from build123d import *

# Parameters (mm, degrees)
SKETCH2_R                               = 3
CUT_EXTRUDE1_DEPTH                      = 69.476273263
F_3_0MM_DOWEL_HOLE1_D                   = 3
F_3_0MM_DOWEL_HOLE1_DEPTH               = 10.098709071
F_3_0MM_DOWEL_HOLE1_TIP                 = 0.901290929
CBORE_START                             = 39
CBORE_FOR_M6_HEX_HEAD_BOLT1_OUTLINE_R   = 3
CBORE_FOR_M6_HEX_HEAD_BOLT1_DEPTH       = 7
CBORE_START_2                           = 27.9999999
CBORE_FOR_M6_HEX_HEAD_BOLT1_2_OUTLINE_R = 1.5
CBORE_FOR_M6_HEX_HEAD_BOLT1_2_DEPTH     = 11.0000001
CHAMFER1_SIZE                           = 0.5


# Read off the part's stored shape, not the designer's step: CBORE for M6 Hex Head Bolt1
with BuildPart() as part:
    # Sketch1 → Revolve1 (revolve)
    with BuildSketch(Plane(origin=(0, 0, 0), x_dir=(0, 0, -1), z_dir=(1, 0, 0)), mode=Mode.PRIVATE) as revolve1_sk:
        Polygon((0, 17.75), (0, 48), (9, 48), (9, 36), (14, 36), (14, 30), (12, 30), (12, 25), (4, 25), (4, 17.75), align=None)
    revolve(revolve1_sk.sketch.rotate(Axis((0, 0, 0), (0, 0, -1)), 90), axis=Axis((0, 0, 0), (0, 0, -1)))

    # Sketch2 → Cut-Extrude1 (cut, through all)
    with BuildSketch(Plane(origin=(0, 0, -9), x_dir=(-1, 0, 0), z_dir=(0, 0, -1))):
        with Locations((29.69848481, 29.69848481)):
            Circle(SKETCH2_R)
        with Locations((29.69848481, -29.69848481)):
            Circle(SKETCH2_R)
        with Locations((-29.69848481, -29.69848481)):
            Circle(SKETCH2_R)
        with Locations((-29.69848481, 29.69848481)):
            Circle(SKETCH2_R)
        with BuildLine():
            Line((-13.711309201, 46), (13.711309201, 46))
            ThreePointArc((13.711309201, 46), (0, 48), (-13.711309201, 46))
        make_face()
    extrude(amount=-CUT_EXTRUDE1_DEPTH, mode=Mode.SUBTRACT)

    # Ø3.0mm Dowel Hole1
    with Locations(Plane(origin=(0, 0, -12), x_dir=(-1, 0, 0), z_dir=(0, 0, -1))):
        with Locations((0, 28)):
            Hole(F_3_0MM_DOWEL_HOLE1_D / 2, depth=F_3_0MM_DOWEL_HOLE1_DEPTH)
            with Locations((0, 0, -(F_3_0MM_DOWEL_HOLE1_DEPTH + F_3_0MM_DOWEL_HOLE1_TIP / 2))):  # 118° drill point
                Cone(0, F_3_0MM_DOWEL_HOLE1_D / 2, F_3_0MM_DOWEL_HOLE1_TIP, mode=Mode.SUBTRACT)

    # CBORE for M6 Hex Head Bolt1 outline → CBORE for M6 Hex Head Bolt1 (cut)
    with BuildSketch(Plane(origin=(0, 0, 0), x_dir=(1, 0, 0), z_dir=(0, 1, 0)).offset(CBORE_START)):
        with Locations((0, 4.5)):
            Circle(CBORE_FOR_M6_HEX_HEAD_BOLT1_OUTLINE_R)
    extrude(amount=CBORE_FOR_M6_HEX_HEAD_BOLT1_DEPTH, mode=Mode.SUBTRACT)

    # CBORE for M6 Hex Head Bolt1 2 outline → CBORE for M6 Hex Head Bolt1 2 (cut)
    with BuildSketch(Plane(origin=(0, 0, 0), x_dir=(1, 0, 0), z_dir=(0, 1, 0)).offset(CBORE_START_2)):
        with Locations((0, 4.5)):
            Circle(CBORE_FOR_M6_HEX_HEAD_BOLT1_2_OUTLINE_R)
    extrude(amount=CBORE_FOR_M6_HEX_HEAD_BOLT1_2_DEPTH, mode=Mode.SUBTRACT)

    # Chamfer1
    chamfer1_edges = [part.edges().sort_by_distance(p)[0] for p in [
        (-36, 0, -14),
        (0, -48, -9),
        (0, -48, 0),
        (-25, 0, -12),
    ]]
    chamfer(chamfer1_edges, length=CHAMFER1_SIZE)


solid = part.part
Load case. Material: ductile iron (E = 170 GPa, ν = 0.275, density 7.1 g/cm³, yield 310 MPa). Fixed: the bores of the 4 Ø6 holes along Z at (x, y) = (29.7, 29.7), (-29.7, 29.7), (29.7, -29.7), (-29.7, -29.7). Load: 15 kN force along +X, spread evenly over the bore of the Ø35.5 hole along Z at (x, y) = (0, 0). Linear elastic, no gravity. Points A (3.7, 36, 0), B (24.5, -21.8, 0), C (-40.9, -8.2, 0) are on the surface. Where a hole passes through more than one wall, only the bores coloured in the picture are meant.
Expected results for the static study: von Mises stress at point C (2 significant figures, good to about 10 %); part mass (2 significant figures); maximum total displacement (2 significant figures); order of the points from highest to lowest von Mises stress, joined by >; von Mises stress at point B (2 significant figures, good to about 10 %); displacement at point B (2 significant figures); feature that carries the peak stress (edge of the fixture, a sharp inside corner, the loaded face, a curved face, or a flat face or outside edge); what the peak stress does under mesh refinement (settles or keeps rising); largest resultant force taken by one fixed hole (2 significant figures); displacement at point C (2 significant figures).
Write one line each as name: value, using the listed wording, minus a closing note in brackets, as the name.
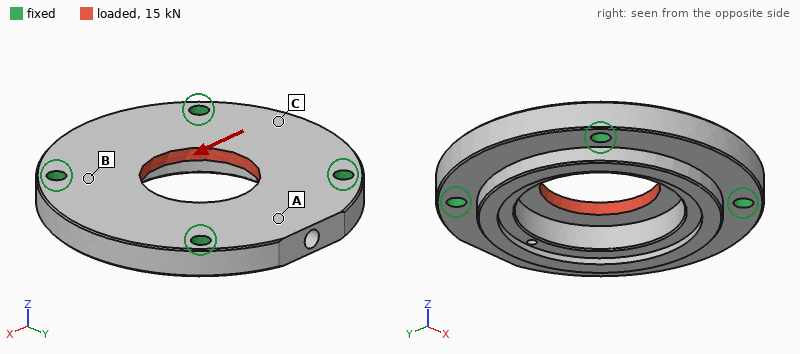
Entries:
von Mises stress at point C: 12 MPa
part mass: 410 g
maximum total displacement: 8.8 µm
order of the points from highest to lowest von Mises stress, joined by >: B > C > A
von Mises stress at point B: 33 MPa
displacement at point B: 2.1 µm
feature that carries the peak stress: edge of the fixture
what the peak stress does under mesh refinement: keeps rising
largest resultant force taken by one fixed hole: 3.8 kN
displacement at point C: 5.0 µm
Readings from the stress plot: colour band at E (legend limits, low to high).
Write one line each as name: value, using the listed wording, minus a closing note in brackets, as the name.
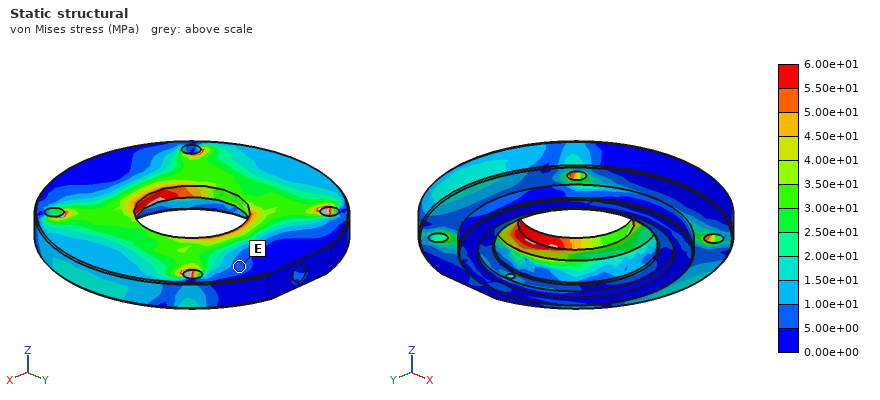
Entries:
colour band at E: 5.00e+00 to 1.00e+01 MPa
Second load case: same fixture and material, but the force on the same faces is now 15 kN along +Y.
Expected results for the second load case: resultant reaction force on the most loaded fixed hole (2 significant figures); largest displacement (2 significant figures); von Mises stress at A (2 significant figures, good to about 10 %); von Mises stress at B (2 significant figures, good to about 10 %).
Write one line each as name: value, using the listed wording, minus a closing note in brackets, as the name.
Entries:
resultant reaction force on the most loaded fixed hole: 3.8 kN
largest displacement: 9.3 µm
von Mises stress at A: 18 MPa
von Mises stress at B: 31 MPa
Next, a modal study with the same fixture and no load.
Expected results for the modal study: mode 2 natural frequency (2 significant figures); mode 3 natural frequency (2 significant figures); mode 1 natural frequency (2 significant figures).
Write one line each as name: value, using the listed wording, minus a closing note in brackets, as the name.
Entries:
mode 2 natural frequency: 11 kHz
mode 3 natural frequency: 11 kHz
mode 1 natural frequency: 9800 Hz
